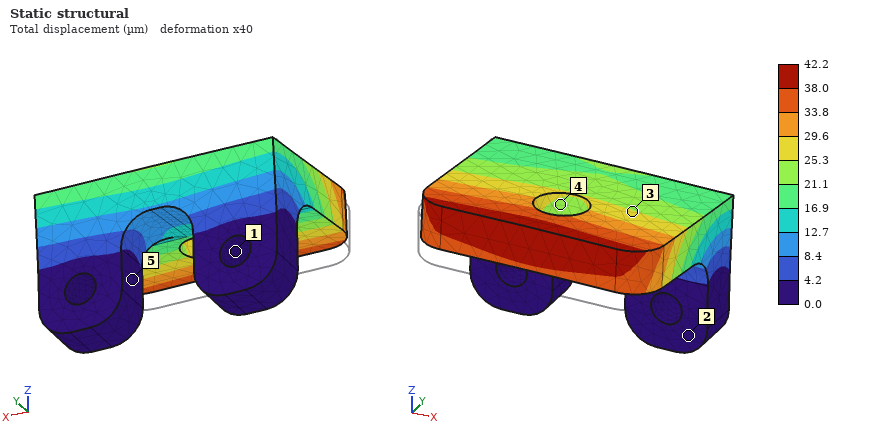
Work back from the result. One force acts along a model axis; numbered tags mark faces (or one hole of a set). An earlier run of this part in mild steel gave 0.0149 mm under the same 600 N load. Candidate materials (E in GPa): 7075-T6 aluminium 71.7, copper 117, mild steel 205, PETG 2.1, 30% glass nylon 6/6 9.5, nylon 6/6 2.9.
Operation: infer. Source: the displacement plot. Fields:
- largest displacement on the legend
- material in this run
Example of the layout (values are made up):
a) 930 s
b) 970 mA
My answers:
a) 42.2 µm
b) 7075-T6 aluminium
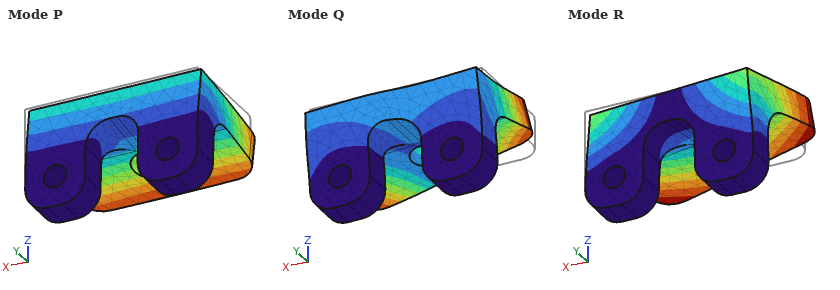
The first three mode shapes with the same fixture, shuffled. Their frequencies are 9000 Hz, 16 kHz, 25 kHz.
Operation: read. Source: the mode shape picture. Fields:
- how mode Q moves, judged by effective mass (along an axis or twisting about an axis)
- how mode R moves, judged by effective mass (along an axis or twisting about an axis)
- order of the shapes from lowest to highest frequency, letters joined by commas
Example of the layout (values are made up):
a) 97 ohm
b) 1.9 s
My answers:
a) along X
b) along X
c) P, R, Q
